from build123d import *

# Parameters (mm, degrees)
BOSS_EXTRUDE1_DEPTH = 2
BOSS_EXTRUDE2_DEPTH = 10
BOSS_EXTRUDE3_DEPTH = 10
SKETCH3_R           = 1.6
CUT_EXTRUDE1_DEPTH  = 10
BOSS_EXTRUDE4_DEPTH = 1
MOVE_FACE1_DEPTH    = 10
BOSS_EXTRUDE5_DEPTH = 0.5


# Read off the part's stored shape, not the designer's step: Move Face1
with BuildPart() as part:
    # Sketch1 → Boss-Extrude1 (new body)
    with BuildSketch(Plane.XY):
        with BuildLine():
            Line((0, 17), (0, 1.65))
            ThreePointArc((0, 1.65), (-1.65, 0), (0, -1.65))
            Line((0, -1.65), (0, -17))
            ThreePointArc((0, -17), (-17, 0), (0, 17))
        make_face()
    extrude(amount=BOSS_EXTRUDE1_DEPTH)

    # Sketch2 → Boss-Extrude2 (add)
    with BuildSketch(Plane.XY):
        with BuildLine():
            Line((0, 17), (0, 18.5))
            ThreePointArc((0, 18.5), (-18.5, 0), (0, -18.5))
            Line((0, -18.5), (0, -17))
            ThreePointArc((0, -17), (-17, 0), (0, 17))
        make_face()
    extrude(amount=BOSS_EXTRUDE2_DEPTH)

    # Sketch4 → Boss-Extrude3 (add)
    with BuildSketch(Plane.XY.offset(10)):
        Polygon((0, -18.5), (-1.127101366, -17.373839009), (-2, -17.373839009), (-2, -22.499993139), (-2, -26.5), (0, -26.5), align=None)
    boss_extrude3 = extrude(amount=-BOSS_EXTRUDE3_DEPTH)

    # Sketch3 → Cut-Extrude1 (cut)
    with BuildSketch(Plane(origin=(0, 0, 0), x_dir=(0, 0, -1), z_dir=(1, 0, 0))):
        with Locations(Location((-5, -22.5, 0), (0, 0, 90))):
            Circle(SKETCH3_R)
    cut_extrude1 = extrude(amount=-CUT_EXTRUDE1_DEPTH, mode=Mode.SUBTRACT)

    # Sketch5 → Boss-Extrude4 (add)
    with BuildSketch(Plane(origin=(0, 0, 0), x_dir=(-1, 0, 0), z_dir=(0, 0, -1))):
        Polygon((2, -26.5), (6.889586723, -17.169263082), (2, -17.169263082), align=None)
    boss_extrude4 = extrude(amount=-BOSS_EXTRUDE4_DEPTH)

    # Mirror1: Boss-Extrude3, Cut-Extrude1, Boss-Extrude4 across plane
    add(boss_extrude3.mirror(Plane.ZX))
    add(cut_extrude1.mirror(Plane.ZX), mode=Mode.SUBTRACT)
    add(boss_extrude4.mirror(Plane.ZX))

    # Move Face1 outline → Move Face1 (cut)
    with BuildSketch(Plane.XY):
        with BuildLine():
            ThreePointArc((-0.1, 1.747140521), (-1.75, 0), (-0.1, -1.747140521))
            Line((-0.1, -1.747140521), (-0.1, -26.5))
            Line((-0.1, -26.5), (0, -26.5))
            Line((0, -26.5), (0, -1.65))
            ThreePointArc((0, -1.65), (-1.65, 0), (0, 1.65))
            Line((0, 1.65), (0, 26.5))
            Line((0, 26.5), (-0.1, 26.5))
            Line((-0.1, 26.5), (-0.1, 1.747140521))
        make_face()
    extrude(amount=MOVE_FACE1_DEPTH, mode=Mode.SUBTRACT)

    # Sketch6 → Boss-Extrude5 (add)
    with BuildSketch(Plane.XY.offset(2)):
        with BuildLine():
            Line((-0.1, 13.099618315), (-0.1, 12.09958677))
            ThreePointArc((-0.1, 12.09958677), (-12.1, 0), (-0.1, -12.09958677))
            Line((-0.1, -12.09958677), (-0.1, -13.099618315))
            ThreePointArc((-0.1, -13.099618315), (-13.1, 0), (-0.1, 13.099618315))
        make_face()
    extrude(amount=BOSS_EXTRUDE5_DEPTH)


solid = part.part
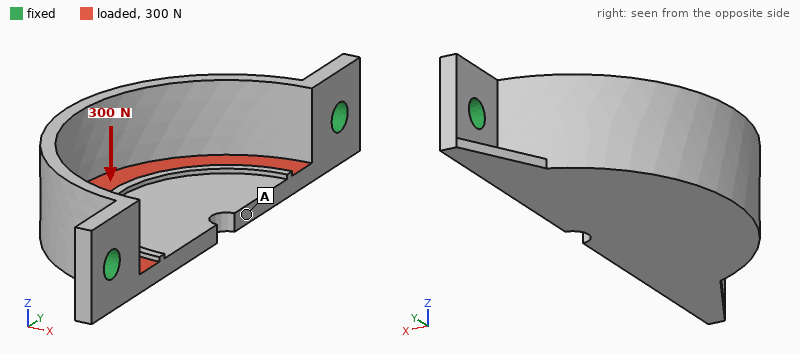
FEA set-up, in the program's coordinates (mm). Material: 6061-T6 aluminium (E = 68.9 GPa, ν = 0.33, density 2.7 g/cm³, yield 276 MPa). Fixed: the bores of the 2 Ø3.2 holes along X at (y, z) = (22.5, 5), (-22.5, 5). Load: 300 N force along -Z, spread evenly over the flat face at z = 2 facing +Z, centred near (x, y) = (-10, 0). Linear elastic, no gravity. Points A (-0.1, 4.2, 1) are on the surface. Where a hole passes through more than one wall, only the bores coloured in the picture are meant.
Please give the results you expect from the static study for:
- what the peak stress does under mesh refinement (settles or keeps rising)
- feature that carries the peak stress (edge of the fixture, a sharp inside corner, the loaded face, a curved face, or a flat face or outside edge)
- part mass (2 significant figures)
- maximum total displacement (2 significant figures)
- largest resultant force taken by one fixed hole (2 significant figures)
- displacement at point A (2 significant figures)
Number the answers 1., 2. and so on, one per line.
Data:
1. keeps rising
2. edge of the fixture
3. 5.6 g
4. 0.11 mm
5. 160 N
6. 0.023 mm
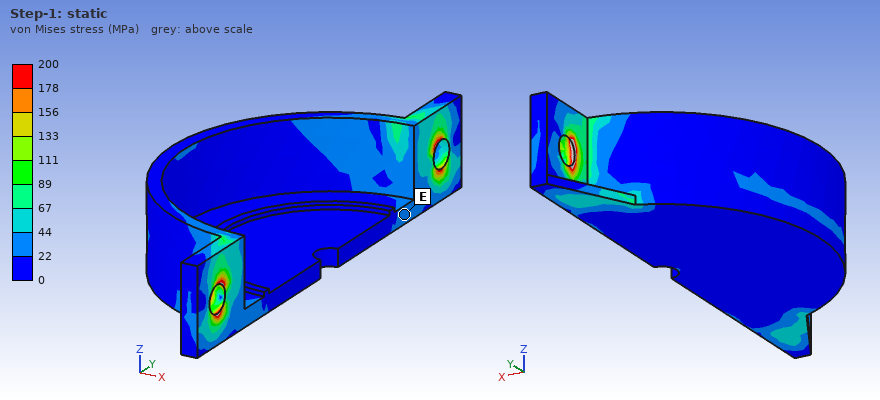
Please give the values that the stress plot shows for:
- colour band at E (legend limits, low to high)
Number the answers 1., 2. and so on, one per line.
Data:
1. 22 to 44 MPa
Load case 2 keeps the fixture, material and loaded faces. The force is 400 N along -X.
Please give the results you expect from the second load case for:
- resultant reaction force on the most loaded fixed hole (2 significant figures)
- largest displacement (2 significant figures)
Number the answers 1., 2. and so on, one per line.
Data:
1. 240 N
2. 39 µm
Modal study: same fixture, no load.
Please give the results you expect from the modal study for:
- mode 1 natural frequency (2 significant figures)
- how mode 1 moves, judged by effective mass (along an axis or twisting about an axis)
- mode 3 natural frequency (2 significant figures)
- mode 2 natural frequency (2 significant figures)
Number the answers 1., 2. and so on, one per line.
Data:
1. 4700 Hz
2. along Z
3. 11 kHz
4. 10 kHz
